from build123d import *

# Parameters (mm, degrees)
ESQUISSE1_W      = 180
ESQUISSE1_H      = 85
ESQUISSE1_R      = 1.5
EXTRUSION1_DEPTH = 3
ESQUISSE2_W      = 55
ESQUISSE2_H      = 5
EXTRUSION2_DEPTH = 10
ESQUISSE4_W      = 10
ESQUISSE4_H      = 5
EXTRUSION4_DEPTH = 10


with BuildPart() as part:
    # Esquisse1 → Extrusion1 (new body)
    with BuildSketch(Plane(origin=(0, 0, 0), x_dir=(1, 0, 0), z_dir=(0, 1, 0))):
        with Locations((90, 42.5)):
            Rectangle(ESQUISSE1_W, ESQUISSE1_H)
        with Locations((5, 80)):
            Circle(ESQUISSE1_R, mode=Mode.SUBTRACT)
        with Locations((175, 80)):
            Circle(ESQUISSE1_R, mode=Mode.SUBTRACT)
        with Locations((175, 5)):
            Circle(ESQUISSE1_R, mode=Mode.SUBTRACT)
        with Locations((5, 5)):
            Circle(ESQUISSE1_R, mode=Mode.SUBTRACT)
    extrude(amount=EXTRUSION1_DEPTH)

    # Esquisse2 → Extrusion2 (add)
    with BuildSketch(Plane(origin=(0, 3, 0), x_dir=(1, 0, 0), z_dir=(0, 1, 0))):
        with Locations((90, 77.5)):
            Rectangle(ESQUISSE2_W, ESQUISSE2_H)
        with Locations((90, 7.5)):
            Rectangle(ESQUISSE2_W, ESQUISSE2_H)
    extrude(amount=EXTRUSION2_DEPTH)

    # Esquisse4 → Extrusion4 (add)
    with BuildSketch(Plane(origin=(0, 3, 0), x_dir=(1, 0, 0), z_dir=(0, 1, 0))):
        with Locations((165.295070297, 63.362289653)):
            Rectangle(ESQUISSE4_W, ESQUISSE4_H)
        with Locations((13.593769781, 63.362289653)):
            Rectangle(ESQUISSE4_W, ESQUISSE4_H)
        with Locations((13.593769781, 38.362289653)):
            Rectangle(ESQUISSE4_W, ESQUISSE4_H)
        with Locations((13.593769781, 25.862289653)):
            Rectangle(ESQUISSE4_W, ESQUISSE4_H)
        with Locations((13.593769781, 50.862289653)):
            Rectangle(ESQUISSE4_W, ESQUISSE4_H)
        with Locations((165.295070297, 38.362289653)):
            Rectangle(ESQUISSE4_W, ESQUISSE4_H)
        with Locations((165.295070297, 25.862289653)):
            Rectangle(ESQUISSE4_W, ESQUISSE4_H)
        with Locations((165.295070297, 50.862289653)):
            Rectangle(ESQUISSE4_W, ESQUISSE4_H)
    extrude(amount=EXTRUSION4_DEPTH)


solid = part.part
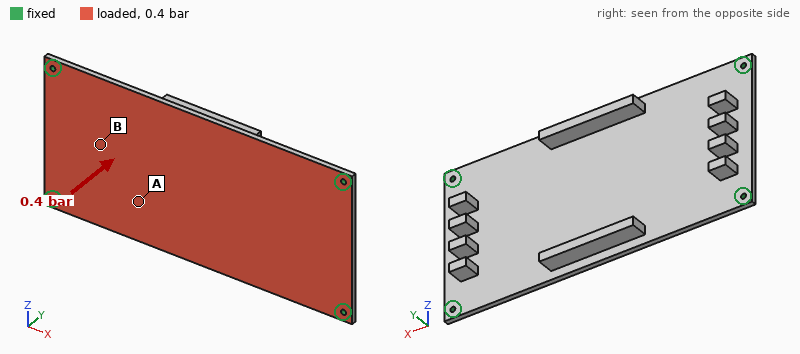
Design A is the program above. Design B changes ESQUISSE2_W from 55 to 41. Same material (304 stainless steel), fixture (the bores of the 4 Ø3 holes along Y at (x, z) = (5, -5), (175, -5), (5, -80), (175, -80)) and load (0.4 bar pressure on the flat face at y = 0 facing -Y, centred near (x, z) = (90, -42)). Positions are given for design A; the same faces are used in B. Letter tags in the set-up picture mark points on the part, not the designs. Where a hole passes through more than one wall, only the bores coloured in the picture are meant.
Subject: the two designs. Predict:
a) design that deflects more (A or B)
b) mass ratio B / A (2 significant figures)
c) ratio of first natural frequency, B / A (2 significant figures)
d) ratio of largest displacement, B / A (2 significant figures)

B
0.97
0.93
1.2
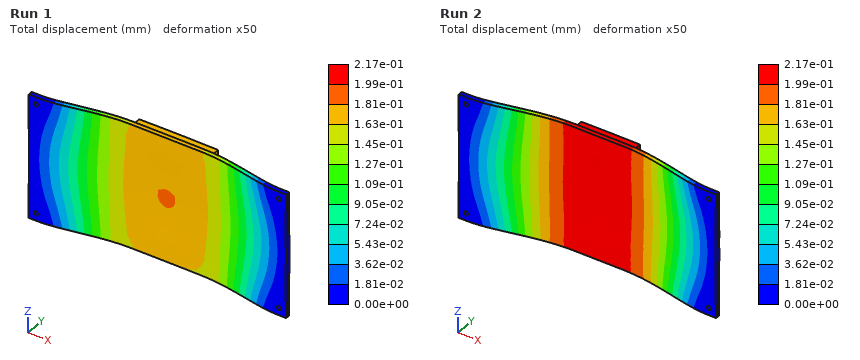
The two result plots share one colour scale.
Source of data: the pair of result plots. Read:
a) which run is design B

Run 2
